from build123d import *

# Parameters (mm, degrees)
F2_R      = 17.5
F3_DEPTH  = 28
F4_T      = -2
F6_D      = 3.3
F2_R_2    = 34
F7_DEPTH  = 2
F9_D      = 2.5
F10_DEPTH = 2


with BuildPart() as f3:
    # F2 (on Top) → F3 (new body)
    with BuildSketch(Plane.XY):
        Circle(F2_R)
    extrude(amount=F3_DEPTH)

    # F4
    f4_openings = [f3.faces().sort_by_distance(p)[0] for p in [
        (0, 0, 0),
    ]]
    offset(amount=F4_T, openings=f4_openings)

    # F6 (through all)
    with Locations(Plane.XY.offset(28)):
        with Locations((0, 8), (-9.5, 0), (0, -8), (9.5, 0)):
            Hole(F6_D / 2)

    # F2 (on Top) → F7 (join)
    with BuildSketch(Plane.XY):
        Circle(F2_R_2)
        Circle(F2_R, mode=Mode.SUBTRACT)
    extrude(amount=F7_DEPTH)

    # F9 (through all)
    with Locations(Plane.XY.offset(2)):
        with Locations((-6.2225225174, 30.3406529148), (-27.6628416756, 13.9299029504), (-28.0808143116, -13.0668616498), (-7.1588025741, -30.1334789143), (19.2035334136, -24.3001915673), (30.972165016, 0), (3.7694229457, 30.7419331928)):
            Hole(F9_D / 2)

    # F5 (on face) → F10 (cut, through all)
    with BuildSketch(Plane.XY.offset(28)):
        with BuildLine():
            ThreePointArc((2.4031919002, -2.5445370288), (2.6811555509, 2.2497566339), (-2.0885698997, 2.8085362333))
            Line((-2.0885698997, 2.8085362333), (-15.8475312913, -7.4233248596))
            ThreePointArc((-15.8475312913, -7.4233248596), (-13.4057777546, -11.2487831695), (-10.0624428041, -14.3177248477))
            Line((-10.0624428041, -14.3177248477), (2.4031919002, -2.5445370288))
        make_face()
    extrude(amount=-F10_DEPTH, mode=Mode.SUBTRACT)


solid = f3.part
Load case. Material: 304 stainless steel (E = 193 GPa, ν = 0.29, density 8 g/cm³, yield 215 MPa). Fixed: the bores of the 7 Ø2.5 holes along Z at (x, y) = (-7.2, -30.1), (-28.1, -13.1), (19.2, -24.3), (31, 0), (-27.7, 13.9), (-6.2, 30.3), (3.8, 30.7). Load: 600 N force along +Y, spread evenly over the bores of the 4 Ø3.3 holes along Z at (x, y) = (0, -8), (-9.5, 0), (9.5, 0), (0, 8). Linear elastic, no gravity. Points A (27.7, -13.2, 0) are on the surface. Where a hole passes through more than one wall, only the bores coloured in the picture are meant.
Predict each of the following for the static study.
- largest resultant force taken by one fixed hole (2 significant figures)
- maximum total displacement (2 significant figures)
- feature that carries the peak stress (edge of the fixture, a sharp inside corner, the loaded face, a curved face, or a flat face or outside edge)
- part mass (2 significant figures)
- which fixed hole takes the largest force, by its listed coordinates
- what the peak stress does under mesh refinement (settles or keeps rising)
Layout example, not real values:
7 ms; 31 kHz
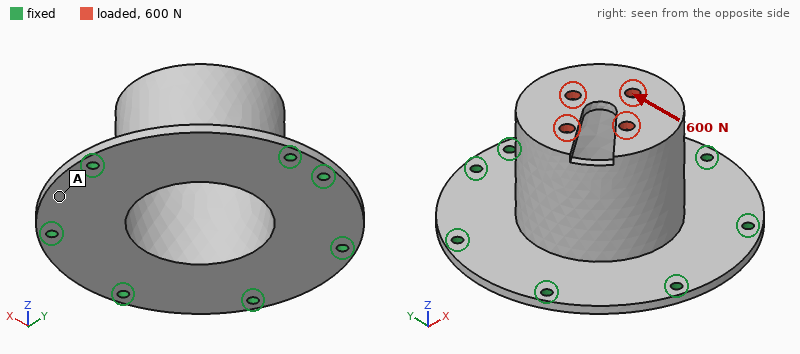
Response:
230 N; 41 µm; edge of the fixture; 98 g; (-7.2, -30.1); keeps rising
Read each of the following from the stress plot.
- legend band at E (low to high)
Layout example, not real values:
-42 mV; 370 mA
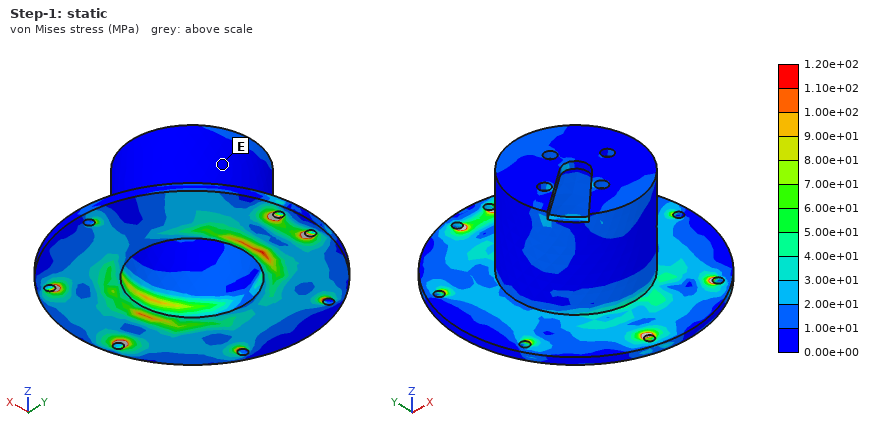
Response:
0.00e+00 to 1.00e+01 MPa
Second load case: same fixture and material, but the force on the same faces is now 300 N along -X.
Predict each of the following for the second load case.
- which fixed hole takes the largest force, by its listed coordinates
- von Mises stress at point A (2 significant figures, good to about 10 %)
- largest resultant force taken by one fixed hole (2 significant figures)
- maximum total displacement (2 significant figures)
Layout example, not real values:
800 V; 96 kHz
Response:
(31, 0); 11 MPa; 140 N; 22 µm
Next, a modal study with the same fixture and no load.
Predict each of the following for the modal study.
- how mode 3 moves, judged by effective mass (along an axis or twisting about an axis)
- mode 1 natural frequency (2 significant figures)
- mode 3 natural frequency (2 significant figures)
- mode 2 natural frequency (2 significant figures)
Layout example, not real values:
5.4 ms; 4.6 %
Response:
along Z; 3300 Hz; 4100 Hz; 3700 Hz
